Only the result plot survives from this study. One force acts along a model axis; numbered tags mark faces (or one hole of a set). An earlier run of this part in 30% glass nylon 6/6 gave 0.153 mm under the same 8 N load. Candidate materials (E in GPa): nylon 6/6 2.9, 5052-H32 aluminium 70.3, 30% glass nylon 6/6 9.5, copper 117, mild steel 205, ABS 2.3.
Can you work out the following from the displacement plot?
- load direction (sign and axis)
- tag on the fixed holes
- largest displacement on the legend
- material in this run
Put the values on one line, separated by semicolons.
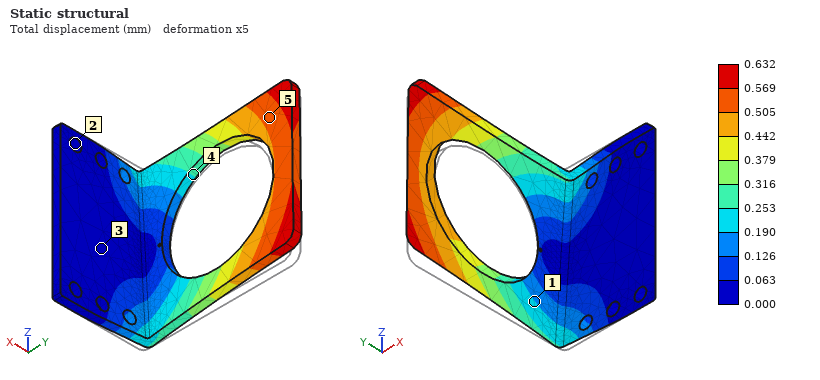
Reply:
+Z; 2; 0.632 mm; ABS
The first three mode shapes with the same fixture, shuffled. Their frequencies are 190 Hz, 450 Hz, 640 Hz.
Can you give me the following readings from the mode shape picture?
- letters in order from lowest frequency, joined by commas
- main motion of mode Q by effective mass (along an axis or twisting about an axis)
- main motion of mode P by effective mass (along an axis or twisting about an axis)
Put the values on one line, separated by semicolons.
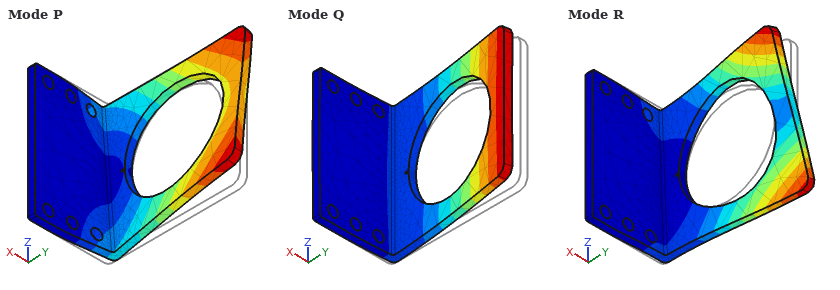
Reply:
Q, P, R; along X; along Z
